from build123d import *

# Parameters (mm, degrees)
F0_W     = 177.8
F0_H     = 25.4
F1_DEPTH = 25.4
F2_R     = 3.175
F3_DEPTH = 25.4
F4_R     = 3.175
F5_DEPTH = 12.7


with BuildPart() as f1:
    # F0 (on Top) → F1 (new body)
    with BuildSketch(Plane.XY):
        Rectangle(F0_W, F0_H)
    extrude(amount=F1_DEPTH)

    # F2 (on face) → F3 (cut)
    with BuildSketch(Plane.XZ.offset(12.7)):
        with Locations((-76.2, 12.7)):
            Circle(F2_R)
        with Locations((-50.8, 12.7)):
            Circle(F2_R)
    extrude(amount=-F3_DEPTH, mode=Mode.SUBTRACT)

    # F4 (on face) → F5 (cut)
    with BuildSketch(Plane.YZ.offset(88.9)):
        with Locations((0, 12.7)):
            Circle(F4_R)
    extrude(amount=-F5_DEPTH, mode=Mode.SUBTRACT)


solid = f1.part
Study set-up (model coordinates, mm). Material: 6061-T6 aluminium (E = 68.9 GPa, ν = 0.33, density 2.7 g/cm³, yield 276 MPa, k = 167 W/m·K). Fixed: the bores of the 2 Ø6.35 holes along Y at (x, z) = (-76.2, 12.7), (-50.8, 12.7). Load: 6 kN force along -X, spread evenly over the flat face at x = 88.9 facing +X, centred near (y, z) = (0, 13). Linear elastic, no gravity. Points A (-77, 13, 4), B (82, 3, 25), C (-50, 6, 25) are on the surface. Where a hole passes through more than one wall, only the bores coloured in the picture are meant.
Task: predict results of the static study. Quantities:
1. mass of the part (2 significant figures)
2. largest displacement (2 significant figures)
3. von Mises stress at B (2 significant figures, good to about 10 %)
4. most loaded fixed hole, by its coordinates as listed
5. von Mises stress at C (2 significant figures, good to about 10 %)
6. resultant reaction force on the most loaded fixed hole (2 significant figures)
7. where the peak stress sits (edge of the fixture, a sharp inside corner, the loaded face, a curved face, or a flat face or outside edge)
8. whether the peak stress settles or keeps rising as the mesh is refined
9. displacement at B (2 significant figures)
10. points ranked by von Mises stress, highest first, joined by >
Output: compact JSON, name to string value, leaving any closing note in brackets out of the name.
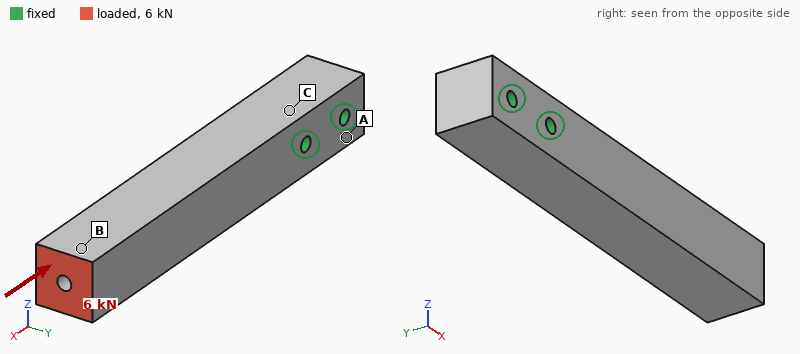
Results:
{"mass of the part": "300 g", "largest displacement": "19 µm", "von Mises stress at B": "9.7 MPa", "most loaded fixed hole, by its coordinates as listed": "(-50.8, 12.7)", "von Mises stress at C": "5.1 MPa", "resultant reaction force on the most loaded fixed hole": "5.2 kN", "where the peak stress sits": "edge of the fixture", "whether the peak stress settles or keeps rising as the mesh is refined": "keeps rising", "displacement at B": "18 µm", "points ranked by von Mises stress, highest first, joined by >": "B > C > A"}
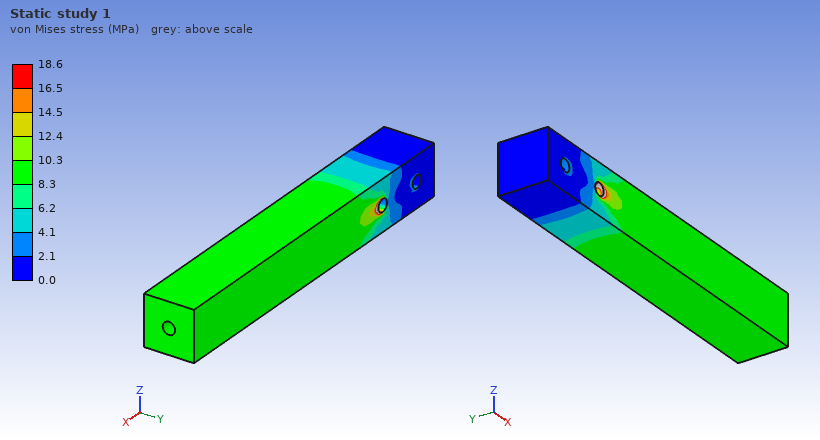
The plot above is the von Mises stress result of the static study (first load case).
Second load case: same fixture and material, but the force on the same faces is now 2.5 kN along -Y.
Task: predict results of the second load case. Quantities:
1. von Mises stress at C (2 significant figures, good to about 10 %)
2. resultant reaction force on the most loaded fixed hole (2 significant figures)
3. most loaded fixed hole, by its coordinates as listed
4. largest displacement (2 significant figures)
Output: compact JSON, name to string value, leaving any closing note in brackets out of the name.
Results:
{"von Mises stress at C": "43 MPa", "resultant reaction force on the most loaded fixed hole": "4.8 kN", "most loaded fixed hole, by its coordinates as listed": "(-50.8, 12.7)", "largest displacement": "1.0 mm"}
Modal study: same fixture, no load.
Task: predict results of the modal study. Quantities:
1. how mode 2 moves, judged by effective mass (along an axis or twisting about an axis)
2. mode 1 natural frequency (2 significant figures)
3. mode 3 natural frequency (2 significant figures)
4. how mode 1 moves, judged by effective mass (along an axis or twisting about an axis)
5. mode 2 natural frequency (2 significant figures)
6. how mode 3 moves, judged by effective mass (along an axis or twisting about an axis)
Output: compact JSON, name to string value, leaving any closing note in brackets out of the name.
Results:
{"how mode 2 moves, judged by effective mass": "along Y", "mode 1 natural frequency": "930 Hz", "mode 3 natural frequency": "5100 Hz", "how mode 1 moves, judged by effective mass": "along Z", "mode 2 natural frequency": "1000 Hz", "how mode 3 moves, judged by effective mass": "twisting about X"}
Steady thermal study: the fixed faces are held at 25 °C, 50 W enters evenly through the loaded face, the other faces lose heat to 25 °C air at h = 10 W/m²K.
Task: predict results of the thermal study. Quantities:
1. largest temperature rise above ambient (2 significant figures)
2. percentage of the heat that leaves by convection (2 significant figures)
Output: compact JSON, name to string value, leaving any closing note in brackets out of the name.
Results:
{"largest temperature rise above ambient": "61 K", "percentage of the heat that leaves by convection": "8.9 %"}
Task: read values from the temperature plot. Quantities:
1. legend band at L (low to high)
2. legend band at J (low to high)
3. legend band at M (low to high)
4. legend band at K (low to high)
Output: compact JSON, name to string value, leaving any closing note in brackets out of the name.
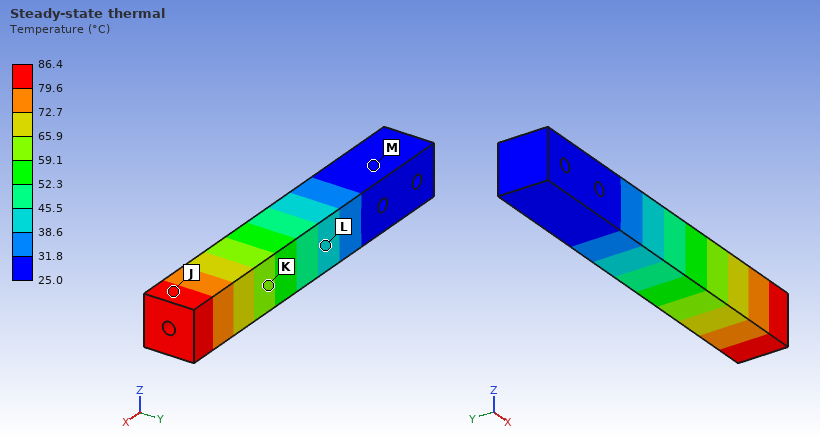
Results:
{"legend band at L": "38.6 to 45.5 °C", "legend band at J": "79.6 to 86.4 °C", "legend band at M": "25.0 to 31.8 °C", "legend band at K": "59.1 to 65.9 °C"}
